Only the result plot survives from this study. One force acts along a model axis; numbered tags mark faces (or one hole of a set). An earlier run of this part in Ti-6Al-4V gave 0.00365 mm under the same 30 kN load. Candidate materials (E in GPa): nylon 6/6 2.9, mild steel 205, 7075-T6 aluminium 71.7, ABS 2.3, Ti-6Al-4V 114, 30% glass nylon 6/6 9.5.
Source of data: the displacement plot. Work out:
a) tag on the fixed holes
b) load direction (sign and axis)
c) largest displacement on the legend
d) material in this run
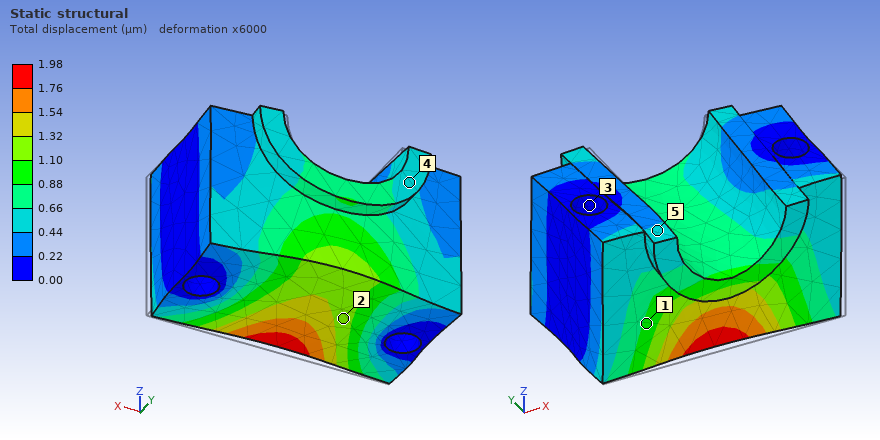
3
+Y
1.98 µm
mild steel
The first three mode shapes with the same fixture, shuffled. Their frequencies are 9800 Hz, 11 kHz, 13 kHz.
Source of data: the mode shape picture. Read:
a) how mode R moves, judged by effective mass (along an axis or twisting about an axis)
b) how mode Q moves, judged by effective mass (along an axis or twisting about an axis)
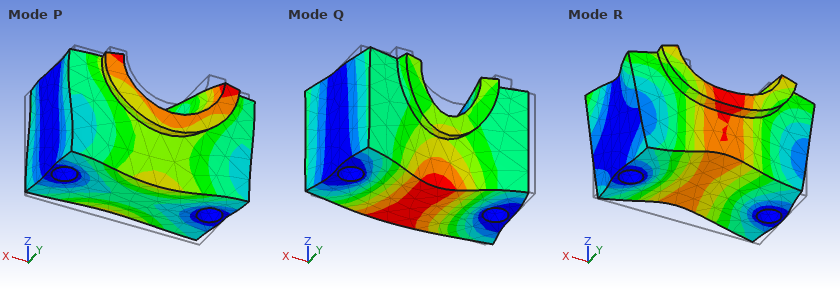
along Z
along Y
